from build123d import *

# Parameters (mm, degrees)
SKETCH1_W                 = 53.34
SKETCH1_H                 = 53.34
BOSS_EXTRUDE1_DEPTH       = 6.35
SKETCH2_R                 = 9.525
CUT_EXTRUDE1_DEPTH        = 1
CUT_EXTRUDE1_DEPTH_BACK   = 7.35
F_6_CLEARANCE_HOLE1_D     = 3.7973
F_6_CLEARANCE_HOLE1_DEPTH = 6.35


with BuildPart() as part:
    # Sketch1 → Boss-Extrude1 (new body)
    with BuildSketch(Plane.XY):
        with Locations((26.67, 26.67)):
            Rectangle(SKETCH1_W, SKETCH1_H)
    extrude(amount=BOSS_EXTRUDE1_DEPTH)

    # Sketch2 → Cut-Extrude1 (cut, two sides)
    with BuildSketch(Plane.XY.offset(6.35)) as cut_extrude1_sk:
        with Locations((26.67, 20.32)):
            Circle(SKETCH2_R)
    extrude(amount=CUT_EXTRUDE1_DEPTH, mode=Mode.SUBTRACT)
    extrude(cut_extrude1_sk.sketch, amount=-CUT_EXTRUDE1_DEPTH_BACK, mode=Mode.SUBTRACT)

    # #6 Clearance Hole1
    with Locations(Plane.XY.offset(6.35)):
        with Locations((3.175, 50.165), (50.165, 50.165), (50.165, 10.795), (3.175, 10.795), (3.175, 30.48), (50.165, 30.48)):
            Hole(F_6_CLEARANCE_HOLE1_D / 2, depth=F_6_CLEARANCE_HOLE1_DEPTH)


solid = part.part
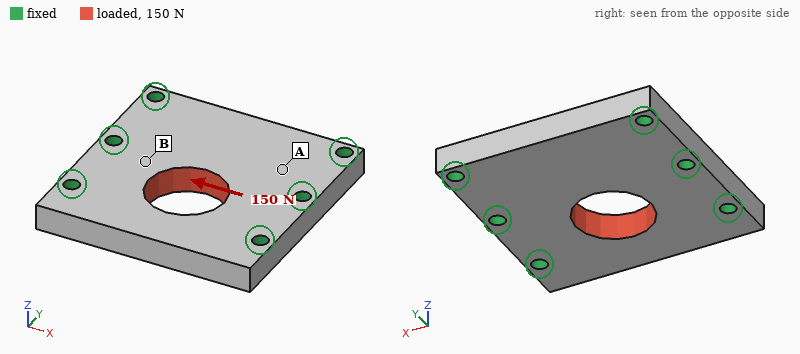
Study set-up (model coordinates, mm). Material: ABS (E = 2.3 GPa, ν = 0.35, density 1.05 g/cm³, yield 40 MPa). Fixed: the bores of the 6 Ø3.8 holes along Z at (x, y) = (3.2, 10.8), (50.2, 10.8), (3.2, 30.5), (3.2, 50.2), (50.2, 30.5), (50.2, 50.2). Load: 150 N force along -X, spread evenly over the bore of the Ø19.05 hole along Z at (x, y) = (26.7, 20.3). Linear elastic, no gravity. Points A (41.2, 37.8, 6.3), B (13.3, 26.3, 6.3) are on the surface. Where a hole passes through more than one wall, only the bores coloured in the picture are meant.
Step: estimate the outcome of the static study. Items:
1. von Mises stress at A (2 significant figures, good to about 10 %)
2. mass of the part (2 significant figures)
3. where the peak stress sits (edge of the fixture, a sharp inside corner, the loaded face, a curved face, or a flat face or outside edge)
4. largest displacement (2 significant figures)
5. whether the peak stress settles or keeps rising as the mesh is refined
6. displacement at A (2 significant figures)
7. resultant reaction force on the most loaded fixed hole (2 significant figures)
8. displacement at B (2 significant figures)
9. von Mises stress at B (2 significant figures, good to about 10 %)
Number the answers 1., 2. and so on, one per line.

1. 0.13 MPa
2. 17 g
3. edge of the fixture
4. 4.4 µm
5. keeps rising
6. 1.0 µm
7. 39 N
8. 2.0 µm
9. 0.39 MPa
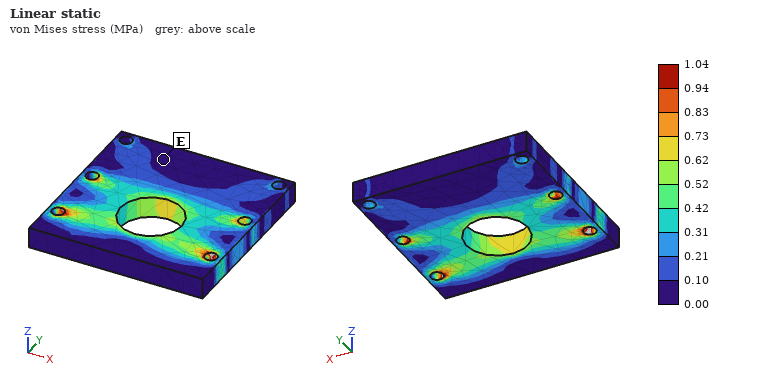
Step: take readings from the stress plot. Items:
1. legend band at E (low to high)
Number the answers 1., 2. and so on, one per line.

1. 0.00 to 0.10 MPa
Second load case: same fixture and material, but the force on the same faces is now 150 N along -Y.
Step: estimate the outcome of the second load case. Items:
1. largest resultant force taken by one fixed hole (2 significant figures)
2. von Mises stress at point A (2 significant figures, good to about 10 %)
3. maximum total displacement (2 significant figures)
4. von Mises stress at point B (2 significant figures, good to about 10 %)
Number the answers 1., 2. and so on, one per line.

1. 35 N
2. 0.39 MPa
3. 10 µm
4. 0.54 MPa
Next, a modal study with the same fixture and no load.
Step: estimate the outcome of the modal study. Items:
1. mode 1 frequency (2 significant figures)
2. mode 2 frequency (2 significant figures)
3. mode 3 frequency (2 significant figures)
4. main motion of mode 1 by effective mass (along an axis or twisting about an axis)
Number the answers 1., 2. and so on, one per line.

1. 3800 Hz
2. 4100 Hz
3. 6400 Hz
4. along Z
